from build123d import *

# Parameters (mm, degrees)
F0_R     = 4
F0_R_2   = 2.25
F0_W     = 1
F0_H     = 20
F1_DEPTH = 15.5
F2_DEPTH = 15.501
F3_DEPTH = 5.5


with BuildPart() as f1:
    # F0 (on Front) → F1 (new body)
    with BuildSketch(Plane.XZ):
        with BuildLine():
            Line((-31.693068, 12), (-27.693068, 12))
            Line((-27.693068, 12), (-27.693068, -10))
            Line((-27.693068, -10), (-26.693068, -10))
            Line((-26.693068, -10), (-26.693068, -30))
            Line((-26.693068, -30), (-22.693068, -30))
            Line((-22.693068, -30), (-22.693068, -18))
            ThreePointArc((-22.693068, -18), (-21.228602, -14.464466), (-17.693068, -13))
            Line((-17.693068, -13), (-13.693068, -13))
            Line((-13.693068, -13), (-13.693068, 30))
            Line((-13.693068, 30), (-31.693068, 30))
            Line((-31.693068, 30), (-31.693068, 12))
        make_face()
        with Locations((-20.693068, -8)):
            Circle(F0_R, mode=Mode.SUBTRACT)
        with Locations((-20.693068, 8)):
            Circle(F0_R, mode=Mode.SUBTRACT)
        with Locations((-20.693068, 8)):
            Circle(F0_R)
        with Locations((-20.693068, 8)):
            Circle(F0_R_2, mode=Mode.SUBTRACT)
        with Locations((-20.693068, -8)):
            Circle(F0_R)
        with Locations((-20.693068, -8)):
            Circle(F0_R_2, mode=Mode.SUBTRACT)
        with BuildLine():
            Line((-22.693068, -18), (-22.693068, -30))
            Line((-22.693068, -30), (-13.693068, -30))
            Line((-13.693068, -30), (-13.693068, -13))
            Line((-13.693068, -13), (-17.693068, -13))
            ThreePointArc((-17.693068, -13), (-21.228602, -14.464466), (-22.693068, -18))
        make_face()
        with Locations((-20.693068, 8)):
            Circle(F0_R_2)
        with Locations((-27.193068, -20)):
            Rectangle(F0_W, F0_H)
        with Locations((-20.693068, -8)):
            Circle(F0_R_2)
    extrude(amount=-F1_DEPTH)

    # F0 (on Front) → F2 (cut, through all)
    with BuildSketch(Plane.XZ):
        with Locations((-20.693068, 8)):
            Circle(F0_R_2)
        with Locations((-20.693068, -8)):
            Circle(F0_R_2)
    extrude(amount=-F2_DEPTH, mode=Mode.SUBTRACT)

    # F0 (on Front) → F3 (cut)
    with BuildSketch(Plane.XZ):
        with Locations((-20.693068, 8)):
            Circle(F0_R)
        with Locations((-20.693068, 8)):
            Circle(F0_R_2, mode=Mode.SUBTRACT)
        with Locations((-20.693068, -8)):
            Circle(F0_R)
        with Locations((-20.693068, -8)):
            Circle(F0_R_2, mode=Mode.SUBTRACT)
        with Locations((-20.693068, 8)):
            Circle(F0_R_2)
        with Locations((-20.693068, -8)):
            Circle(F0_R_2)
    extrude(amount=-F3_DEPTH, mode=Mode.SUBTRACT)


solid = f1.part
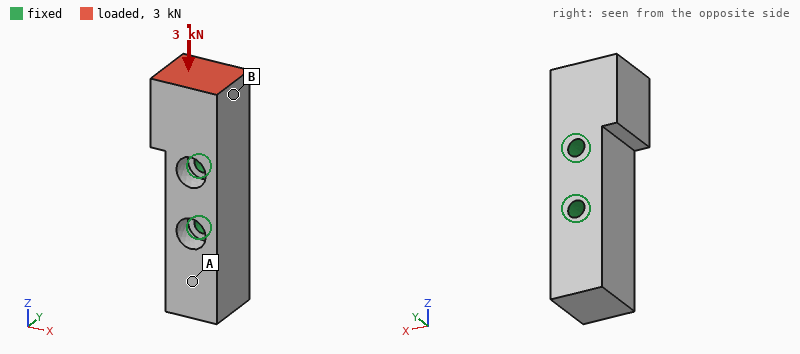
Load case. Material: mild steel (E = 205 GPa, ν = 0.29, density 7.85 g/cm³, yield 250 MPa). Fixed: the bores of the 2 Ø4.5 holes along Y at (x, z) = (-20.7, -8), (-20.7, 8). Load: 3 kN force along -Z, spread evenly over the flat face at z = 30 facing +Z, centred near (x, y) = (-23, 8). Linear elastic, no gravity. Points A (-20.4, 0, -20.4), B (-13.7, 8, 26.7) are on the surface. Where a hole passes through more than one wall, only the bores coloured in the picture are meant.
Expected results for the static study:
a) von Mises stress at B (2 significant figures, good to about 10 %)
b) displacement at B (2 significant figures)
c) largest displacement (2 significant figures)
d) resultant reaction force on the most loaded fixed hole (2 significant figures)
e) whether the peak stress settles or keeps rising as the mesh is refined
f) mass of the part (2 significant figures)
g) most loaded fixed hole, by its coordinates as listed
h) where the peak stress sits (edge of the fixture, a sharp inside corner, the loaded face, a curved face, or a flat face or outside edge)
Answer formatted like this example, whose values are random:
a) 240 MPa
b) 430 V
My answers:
a) 11 MPa
b) 2.3 µm
c) 4.6 µm
d) 2.5 kN
e) keeps rising
f) 100 g
g) (-20.7, 8)
h) edge of the fixture
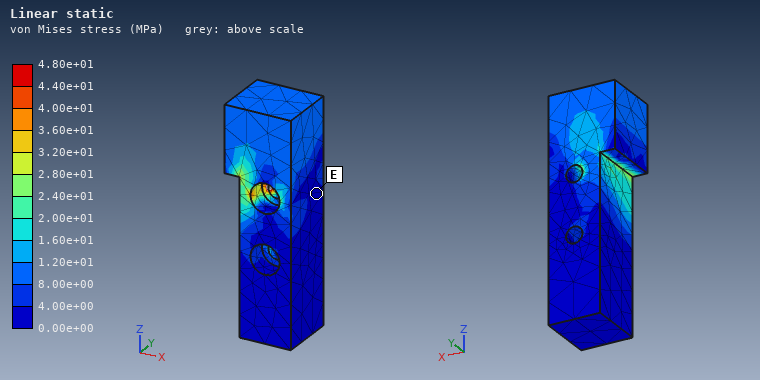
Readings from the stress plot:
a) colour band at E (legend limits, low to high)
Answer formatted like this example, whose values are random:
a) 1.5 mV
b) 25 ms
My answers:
a) 0.00e+00 to 4.00e+00 MPa
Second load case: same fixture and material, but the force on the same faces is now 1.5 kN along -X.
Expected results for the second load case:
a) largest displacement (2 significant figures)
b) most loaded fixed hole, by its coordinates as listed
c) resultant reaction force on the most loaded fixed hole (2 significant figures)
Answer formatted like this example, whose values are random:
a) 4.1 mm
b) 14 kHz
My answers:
a) 16 µm
b) (-20.7, 8)
c) 2.6 kN
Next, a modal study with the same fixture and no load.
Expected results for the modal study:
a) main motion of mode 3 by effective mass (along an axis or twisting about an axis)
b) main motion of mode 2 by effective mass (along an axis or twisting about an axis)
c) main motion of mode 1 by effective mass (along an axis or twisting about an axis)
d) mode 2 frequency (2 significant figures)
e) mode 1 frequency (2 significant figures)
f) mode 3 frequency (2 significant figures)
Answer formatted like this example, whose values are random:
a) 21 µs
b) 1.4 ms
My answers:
a) along X
b) along Y
c) along X
d) 14 kHz
e) 13 kHz
f) 15 kHz
